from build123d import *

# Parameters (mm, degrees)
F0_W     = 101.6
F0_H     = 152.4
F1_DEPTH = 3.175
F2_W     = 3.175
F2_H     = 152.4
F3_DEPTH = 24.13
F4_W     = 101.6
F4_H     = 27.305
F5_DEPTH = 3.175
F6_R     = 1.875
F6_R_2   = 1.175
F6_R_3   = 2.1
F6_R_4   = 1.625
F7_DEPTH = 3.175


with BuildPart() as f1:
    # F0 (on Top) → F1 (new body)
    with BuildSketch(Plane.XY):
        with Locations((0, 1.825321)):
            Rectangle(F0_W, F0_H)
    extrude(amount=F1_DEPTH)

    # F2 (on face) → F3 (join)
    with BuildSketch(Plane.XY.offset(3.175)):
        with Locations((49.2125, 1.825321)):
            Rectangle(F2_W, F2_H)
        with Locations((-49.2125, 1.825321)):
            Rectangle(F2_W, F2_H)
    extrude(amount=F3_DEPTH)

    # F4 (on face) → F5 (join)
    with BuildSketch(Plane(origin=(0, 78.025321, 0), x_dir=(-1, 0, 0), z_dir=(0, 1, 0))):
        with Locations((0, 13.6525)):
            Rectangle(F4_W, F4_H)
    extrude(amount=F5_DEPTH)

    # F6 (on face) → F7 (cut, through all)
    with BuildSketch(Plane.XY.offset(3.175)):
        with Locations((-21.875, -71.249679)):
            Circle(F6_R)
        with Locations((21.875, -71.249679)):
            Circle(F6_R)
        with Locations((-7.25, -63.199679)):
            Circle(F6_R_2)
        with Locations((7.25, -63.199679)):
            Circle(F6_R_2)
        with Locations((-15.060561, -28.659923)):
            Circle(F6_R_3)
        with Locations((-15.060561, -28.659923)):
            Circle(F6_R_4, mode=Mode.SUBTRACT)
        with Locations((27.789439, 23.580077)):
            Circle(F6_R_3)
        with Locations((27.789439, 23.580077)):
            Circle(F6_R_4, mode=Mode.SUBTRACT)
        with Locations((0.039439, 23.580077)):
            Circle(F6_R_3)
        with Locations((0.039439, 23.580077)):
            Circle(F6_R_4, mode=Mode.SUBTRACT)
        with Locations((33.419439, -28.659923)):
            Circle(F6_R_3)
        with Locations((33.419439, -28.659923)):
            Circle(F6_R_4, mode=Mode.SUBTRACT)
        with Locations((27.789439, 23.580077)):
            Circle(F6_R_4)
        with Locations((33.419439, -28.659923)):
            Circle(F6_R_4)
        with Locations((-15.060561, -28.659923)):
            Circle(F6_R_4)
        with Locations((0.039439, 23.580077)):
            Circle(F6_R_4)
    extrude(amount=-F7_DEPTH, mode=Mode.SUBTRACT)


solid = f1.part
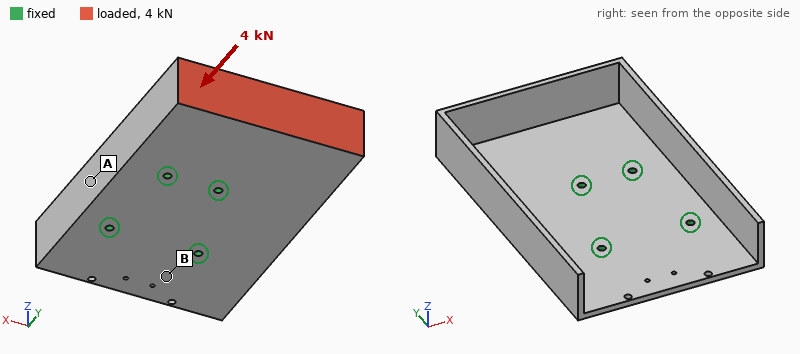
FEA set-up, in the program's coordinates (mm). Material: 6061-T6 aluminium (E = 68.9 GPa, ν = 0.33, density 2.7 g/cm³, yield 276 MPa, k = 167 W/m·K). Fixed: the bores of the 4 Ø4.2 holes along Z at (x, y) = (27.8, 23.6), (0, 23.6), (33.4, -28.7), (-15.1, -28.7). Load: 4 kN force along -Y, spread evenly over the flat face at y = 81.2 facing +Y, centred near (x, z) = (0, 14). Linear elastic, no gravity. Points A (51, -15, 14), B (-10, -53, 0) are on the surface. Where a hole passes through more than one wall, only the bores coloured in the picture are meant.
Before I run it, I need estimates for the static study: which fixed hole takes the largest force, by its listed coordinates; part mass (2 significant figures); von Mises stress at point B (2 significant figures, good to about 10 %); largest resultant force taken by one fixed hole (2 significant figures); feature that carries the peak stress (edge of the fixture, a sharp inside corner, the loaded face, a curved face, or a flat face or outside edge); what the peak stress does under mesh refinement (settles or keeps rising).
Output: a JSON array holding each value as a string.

["(0, 23.6)", "220 g", "36 MPa", "1.6 kN", "edge of the fixture", "keeps rising"]
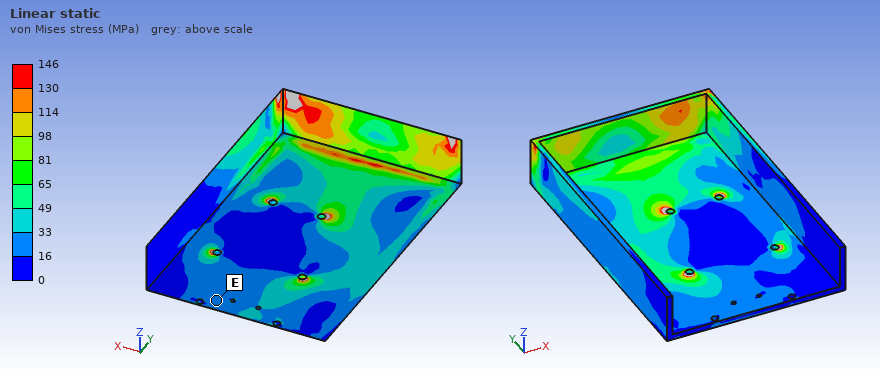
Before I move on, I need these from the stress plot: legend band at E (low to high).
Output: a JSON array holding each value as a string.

["16 to 33 MPa"]
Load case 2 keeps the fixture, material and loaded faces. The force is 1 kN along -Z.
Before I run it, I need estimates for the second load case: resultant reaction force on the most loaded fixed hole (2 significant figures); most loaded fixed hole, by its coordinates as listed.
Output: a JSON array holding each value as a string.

["1.0 kN", "(0, 23.6)"]
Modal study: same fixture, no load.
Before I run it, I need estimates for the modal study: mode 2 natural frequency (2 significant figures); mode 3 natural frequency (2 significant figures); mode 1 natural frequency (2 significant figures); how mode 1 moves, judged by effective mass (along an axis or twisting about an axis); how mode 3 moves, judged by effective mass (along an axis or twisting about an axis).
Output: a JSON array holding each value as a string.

["820 Hz", "990 Hz", "500 Hz", "along Z", "along Z"]
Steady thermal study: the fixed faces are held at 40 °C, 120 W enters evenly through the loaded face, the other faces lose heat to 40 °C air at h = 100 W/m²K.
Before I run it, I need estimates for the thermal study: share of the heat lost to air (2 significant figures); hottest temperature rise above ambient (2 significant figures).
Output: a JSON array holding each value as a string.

["69 %", "78 K"]
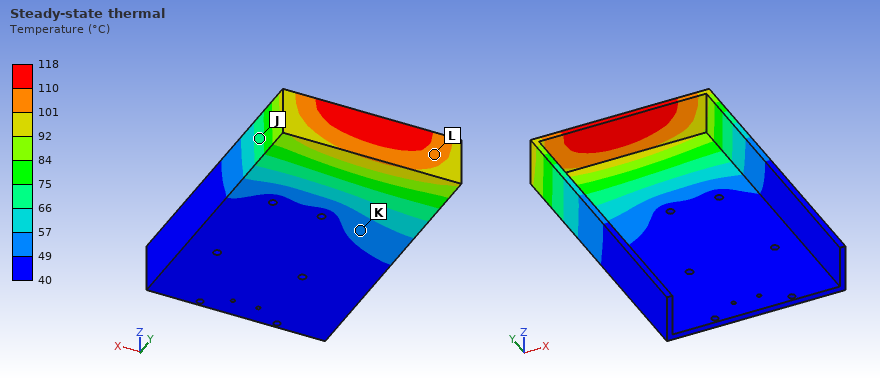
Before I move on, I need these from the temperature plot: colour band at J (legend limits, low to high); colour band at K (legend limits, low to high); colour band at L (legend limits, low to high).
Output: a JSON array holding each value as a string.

["66 to 75 °C", "49 to 57 °C", "101 to 110 °C"]
